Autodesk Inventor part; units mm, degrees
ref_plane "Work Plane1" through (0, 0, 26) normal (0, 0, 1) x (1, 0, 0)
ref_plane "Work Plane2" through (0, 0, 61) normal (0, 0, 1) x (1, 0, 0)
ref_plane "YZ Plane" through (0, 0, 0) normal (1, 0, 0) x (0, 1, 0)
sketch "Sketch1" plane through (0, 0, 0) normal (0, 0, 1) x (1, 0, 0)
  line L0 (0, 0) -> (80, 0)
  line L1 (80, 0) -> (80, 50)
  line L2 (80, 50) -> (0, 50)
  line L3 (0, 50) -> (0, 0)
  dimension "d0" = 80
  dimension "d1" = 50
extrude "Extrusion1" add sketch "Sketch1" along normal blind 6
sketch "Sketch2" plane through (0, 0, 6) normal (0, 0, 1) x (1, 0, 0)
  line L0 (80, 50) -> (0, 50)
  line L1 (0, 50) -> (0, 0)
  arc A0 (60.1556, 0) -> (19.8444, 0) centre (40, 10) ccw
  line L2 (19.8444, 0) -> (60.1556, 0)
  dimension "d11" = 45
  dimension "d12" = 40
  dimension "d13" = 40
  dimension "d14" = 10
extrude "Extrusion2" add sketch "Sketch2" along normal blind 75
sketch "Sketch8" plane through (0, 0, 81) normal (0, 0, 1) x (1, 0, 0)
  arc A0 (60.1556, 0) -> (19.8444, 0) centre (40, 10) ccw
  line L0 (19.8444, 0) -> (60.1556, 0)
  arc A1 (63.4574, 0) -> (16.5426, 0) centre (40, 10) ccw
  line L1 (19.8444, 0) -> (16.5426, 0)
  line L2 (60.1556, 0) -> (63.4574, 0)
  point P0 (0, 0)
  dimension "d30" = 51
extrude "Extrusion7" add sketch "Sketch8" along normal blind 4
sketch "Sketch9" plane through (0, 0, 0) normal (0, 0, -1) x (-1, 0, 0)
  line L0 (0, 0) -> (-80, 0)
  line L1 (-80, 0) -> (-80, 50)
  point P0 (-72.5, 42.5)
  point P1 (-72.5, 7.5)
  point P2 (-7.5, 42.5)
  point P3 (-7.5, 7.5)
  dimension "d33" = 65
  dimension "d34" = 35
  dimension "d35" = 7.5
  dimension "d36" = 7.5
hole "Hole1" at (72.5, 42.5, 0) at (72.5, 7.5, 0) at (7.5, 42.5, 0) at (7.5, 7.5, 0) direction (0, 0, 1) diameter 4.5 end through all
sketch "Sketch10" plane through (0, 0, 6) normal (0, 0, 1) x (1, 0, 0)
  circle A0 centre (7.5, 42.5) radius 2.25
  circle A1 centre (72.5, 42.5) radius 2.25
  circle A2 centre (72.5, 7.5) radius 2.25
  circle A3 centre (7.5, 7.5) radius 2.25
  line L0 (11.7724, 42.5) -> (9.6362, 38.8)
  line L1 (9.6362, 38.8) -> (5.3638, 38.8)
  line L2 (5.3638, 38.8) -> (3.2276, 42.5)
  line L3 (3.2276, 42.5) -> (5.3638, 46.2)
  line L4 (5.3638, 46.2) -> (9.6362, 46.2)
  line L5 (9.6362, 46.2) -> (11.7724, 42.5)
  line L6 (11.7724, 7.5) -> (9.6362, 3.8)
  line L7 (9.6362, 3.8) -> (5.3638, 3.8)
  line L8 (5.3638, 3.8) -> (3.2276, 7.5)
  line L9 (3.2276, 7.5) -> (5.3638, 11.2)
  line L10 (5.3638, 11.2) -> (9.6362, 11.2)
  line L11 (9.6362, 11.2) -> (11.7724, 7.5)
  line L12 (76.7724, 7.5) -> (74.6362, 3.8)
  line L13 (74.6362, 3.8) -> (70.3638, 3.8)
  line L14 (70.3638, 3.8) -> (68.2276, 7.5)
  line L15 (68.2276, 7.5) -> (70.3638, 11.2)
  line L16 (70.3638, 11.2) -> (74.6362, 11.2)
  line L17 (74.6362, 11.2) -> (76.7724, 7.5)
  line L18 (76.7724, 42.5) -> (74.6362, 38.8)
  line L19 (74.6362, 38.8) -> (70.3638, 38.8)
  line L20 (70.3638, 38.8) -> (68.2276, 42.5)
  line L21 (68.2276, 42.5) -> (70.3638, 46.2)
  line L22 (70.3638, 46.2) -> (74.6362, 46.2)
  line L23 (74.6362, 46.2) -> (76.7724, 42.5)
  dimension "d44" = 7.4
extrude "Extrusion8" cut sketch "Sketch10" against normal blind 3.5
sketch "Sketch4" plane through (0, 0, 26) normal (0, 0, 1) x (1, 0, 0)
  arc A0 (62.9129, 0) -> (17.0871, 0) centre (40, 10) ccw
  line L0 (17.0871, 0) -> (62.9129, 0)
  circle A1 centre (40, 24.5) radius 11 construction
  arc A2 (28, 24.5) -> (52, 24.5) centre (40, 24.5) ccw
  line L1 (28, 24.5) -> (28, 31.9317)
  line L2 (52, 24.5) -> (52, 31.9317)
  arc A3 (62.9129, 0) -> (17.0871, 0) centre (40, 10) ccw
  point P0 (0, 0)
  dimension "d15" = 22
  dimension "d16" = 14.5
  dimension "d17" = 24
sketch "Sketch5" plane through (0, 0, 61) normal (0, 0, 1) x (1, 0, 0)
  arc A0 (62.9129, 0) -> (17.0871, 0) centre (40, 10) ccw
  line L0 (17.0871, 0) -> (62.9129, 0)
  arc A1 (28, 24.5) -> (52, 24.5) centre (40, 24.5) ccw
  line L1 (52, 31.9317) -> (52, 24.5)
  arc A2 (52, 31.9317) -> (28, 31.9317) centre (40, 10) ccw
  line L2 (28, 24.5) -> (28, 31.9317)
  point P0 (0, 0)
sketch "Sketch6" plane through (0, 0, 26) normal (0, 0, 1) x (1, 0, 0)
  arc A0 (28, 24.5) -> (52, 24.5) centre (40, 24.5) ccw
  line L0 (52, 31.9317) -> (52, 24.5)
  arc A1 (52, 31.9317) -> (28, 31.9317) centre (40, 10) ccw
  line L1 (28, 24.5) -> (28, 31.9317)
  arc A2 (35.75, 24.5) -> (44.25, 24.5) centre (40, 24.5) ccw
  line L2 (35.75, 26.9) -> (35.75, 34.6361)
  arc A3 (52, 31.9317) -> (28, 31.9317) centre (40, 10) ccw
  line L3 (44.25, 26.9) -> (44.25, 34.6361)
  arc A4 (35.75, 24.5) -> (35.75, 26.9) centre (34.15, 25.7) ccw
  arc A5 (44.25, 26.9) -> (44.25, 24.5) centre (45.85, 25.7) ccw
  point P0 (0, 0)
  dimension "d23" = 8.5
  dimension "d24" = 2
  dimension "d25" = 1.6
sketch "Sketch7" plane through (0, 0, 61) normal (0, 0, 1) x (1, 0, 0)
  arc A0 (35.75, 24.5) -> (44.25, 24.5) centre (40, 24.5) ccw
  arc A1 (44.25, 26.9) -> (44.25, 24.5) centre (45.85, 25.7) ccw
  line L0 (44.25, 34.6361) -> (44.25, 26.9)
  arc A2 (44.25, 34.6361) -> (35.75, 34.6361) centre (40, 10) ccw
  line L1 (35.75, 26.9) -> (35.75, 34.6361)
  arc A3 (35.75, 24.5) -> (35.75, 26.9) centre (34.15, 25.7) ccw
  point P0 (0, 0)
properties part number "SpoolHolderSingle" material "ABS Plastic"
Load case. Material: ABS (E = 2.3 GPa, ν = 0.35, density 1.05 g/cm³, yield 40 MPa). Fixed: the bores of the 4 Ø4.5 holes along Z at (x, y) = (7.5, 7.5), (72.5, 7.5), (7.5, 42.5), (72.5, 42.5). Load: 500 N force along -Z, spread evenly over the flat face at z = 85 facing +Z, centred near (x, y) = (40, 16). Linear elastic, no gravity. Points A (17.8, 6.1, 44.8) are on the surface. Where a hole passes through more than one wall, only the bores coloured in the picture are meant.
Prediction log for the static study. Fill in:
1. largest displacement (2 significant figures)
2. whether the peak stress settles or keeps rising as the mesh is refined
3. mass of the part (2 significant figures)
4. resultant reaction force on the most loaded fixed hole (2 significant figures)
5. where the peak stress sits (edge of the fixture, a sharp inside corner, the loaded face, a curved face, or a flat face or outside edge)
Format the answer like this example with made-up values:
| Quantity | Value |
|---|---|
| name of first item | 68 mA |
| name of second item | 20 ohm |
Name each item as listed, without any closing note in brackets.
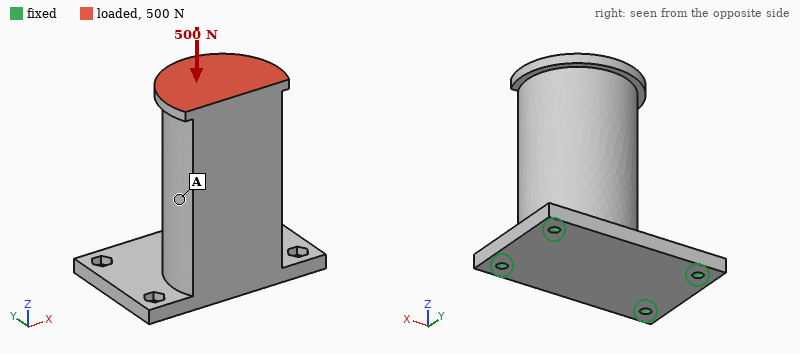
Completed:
| Quantity | Value |
|---|---|
| largest displacement | 0.19 mm |
| whether the peak stress settles or keeps rising as the mesh is refined | keeps rising |
| mass of the part | 130 g |
| resultant reaction force on the most loaded fixed hole | 270 N |
| where the peak stress sits | edge of the fixture |
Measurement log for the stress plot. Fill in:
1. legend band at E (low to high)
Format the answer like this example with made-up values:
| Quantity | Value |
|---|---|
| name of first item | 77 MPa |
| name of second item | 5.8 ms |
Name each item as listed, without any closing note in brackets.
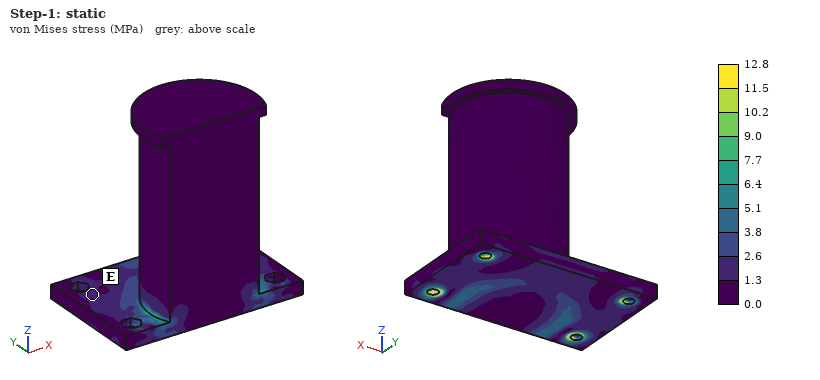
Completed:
| Quantity | Value |
|---|---|
| legend band at E | 1.3 to 2.6 MPa |
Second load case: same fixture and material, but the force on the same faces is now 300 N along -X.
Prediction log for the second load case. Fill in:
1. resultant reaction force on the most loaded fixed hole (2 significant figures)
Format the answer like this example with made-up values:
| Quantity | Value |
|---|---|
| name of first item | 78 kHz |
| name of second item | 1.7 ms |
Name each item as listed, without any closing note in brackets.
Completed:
| Quantity | Value |
|---|---|
| resultant reaction force on the most loaded fixed hole | 390 N |
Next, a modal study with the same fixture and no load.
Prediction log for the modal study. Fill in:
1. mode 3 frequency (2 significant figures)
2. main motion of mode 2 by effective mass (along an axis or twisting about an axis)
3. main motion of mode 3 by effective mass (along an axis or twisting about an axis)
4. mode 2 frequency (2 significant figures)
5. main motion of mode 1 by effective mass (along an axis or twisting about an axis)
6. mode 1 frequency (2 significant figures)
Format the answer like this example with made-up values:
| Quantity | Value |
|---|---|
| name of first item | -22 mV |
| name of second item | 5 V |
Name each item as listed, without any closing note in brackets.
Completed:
| Quantity | Value |
|---|---|
| mode 3 frequency | 930 Hz |
| main motion of mode 2 by effective mass | along X |
| main motion of mode 3 by effective mass | along Z |
| mode 2 frequency | 520 Hz |
| main motion of mode 1 by effective mass | along Y |
| mode 1 frequency | 260 Hz |
